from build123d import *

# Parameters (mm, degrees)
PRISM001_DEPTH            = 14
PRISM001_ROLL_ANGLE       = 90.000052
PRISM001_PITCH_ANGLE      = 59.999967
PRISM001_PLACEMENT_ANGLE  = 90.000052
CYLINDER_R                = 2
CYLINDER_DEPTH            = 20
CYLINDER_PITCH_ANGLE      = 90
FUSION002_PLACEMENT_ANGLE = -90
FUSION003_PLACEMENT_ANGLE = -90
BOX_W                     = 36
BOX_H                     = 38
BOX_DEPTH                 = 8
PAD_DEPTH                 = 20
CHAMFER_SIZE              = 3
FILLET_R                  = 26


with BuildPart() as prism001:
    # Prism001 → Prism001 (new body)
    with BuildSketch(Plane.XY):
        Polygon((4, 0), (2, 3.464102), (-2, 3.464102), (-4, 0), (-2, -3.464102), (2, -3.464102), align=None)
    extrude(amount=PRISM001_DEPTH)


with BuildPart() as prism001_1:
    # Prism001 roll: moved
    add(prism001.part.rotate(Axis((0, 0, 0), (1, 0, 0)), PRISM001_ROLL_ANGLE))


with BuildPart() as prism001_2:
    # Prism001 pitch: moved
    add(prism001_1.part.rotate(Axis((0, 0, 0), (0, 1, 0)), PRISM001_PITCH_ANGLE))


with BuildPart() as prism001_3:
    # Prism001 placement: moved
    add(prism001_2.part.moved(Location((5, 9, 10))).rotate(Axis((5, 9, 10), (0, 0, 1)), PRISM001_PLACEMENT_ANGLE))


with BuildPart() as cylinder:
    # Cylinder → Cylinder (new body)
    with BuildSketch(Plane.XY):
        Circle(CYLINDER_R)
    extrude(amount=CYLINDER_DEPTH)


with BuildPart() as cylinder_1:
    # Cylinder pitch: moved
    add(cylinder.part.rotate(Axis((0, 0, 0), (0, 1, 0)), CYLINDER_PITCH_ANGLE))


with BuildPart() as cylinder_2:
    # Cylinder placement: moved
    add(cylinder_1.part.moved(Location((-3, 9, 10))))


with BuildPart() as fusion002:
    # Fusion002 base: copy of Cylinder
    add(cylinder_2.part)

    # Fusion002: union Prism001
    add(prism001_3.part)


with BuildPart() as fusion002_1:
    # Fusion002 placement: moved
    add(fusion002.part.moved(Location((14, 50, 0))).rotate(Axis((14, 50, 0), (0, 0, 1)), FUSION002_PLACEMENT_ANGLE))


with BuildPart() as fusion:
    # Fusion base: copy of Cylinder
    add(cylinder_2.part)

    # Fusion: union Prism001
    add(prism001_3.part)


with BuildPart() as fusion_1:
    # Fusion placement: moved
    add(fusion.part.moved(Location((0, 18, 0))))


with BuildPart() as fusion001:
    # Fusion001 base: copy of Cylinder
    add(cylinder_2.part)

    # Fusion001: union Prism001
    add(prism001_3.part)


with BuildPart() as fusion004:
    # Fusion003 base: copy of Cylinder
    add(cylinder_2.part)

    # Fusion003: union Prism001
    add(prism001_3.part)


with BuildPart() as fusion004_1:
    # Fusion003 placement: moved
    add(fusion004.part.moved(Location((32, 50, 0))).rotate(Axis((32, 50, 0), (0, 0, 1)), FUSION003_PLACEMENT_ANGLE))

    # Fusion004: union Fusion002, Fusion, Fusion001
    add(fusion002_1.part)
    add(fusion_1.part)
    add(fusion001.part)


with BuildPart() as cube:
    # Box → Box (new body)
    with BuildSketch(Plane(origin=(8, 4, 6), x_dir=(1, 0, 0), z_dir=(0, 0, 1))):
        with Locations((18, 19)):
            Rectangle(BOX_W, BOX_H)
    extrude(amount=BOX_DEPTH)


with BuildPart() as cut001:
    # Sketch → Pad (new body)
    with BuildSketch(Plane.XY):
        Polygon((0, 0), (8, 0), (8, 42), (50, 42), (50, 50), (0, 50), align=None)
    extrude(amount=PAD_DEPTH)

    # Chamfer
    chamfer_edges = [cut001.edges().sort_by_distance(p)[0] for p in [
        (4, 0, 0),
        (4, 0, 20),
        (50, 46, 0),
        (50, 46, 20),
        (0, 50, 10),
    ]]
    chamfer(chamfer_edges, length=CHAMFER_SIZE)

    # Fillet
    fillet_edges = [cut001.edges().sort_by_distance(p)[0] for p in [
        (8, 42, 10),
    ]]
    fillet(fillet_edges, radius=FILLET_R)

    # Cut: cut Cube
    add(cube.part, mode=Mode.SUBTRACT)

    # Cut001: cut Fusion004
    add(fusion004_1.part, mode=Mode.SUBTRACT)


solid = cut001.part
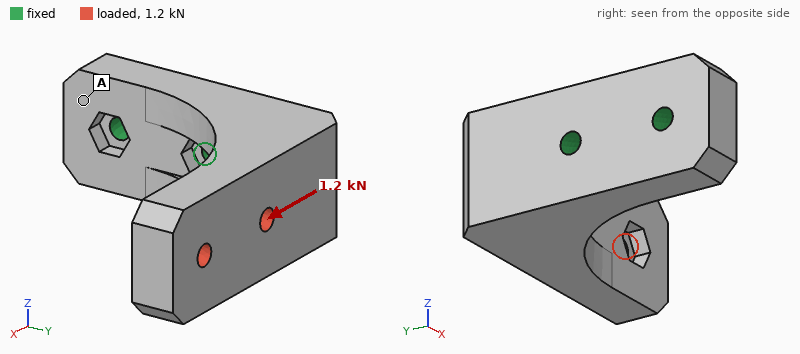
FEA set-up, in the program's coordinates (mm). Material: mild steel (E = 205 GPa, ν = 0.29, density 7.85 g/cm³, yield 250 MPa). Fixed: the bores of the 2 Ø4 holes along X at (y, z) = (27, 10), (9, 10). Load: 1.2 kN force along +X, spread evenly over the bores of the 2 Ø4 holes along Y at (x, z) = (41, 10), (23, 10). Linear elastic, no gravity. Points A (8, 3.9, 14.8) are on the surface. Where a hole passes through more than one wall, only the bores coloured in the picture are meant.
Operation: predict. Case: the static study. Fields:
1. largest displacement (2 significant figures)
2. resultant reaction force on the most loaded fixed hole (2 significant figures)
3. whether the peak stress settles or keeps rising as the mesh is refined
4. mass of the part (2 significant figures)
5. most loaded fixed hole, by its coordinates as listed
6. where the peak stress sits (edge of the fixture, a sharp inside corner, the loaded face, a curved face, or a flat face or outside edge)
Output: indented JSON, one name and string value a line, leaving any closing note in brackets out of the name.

{
  "largest displacement": "55 µm",
  "resultant reaction force on the most loaded fixed hole": "2.3 kN",
  "whether the peak stress settles or keeps rising as the mesh is refined": "keeps rising",
  "mass of the part": "120 g",
  "most loaded fixed hole, by its coordinates as listed": "(27, 10)",
  "where the peak stress sits": "edge of the fixture"
}
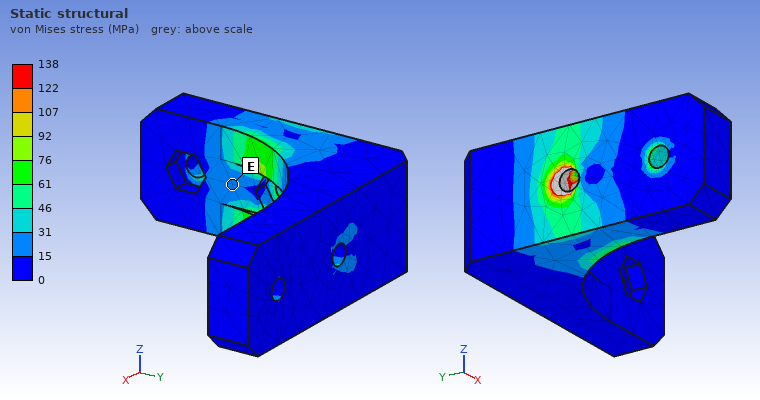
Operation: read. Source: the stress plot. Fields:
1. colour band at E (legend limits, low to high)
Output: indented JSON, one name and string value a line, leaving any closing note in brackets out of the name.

{
  "colour band at E": "15 to 31 MPa"
}
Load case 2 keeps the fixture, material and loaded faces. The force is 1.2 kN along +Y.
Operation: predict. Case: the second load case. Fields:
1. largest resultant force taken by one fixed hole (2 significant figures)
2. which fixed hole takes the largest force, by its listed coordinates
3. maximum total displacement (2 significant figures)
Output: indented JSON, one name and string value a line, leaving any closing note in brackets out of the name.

{
  "largest resultant force taken by one fixed hole": "2.1 kN",
  "which fixed hole takes the largest force, by its listed coordinates": "(9, 10)",
  "maximum total displacement": "0.10 mm"
}
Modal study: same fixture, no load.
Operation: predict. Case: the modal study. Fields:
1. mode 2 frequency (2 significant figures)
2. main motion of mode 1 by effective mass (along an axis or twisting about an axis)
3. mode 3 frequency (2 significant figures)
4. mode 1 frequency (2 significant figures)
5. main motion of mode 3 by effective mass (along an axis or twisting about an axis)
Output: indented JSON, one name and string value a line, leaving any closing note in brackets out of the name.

{
  "mode 2 frequency": "2900 Hz",
  "main motion of mode 1 by effective mass": "along Z",
  "mode 3 frequency": "9300 Hz",
  "mode 1 frequency": "2700 Hz",
  "main motion of mode 3 by effective mass": "along X"
}
